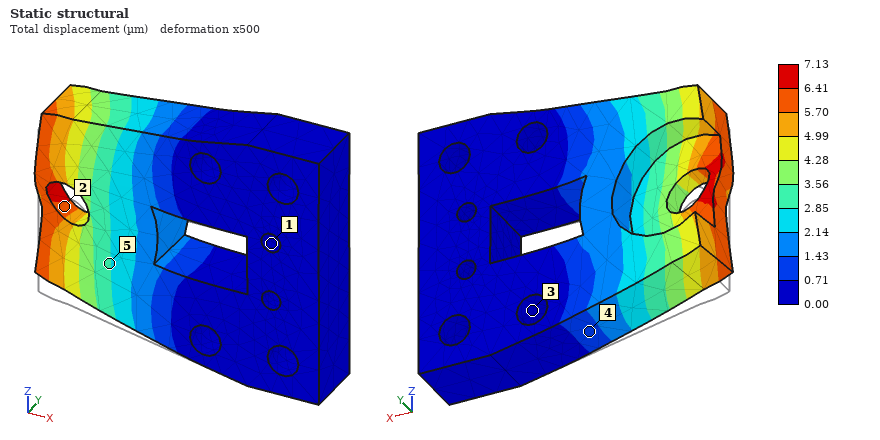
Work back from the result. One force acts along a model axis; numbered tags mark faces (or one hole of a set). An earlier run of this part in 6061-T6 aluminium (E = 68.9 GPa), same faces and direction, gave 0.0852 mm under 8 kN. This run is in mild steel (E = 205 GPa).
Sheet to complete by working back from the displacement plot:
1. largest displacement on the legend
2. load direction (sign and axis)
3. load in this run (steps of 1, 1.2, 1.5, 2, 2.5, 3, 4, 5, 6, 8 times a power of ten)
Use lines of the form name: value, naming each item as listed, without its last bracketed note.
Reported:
largest displacement on the legend: 7.13 µm
load direction: +Z
load in this run: 2 kN
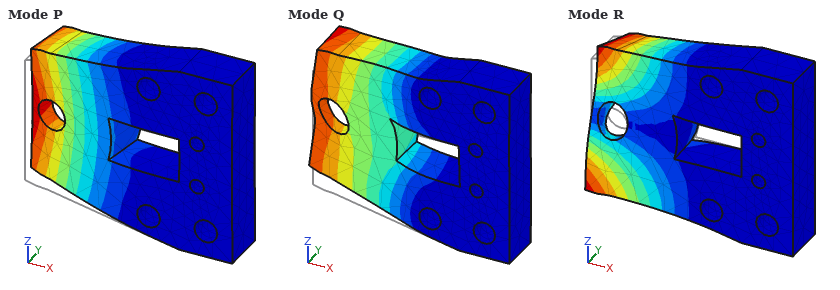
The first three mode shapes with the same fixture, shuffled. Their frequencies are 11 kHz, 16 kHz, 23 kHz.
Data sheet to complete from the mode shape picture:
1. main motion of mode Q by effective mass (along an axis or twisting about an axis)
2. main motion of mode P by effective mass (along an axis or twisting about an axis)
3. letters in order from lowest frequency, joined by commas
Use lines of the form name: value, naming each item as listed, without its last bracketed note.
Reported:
main motion of mode Q by effective mass: along Z
main motion of mode P by effective mass: along Y
letters in order from lowest frequency, joined by commas: P, R, Q
